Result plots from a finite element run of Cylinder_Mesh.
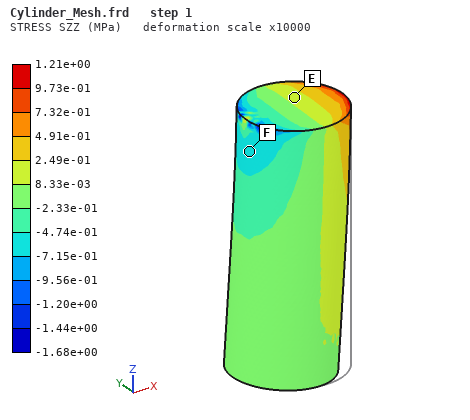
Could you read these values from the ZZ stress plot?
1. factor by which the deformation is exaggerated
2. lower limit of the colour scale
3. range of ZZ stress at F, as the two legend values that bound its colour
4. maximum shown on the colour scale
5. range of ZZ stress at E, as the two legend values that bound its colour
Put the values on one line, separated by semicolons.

10000; -1.68e+00 MPa; -7.15e-01 to -4.74e-01 MPa; 1.21e+00 MPa; 8.33e-03 to 2.49e-01 MPa
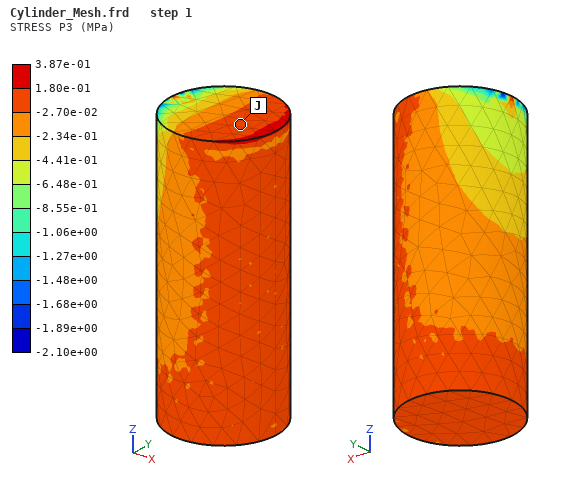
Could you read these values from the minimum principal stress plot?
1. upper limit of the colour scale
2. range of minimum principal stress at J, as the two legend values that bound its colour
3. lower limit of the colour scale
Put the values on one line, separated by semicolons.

3.87e-01 MPa; -2.70e-02 to 1.80e-01 MPa; -2.10e+00 MPa
